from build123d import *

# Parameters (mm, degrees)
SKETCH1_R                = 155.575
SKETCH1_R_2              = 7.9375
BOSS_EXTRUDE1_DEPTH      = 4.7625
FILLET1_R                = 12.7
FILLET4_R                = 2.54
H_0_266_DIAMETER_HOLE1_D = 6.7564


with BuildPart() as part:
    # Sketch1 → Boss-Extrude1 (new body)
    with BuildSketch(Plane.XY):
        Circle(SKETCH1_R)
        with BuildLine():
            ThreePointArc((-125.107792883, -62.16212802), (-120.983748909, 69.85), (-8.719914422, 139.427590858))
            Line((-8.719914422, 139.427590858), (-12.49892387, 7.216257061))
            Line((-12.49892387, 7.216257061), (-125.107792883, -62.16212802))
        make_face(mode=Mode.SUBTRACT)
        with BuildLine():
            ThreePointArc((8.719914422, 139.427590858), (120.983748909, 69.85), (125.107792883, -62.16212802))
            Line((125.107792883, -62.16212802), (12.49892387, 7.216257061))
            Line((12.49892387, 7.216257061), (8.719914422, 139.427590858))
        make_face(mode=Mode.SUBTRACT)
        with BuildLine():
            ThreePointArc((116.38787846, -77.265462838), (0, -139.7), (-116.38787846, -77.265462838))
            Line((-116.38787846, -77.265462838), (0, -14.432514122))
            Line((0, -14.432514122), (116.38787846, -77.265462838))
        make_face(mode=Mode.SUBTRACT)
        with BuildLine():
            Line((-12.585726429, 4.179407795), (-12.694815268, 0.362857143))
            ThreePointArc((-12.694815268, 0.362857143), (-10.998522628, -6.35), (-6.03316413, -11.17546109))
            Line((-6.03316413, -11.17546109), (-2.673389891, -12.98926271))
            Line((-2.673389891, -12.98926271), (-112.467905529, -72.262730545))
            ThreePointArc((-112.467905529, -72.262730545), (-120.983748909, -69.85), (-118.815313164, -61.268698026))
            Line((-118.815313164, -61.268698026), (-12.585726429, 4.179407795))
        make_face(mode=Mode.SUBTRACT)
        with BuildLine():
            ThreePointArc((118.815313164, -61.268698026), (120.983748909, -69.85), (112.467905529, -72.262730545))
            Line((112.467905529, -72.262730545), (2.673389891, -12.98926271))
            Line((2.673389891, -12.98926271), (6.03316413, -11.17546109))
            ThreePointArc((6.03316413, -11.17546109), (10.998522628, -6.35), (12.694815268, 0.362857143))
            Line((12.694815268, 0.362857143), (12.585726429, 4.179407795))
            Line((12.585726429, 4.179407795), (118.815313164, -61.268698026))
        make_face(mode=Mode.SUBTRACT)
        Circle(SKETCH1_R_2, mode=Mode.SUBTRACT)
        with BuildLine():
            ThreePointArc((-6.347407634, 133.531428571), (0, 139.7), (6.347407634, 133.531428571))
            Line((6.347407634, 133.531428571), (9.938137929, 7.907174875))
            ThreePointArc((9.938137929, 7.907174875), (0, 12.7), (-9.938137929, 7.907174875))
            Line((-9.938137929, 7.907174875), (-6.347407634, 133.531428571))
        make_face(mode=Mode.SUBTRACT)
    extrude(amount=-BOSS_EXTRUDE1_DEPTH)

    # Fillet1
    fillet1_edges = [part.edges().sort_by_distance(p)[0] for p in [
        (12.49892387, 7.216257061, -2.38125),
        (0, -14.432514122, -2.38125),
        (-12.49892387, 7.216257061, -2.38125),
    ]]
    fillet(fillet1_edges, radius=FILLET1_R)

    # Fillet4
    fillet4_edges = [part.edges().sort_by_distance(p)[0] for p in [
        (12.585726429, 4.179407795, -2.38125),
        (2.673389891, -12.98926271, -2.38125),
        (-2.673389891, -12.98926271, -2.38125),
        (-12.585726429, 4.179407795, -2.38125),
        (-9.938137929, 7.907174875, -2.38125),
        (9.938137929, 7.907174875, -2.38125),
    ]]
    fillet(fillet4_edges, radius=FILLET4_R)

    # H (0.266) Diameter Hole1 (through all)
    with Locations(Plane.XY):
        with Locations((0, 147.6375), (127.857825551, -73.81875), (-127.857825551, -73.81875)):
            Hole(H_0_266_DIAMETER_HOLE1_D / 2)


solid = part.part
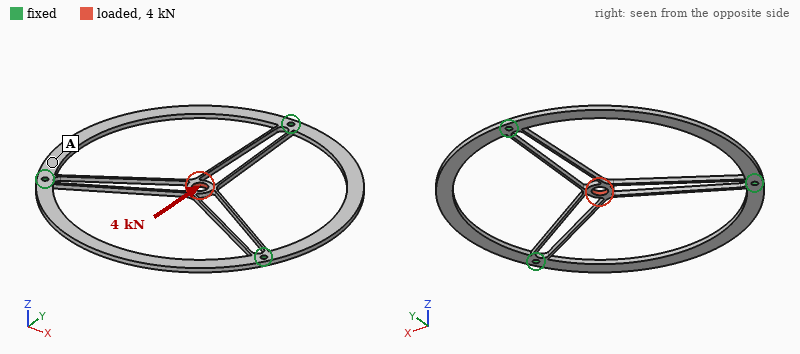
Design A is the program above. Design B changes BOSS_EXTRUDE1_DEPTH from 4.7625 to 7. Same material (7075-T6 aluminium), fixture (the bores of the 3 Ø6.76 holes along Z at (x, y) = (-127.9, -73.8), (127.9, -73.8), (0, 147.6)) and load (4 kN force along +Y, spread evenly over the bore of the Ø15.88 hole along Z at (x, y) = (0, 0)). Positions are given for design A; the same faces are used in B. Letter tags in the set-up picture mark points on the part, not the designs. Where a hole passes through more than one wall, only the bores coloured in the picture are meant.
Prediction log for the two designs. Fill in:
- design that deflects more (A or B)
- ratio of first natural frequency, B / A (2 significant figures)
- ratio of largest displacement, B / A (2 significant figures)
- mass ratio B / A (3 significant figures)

A
1.5
0.68
1.47
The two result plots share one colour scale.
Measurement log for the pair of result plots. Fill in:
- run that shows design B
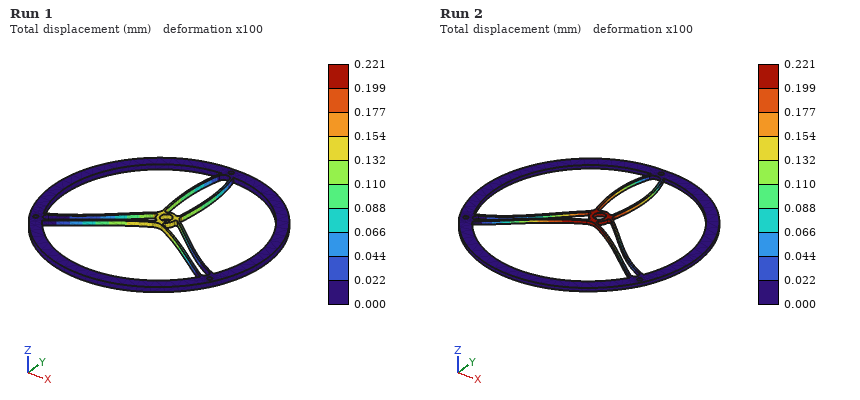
Run 1
